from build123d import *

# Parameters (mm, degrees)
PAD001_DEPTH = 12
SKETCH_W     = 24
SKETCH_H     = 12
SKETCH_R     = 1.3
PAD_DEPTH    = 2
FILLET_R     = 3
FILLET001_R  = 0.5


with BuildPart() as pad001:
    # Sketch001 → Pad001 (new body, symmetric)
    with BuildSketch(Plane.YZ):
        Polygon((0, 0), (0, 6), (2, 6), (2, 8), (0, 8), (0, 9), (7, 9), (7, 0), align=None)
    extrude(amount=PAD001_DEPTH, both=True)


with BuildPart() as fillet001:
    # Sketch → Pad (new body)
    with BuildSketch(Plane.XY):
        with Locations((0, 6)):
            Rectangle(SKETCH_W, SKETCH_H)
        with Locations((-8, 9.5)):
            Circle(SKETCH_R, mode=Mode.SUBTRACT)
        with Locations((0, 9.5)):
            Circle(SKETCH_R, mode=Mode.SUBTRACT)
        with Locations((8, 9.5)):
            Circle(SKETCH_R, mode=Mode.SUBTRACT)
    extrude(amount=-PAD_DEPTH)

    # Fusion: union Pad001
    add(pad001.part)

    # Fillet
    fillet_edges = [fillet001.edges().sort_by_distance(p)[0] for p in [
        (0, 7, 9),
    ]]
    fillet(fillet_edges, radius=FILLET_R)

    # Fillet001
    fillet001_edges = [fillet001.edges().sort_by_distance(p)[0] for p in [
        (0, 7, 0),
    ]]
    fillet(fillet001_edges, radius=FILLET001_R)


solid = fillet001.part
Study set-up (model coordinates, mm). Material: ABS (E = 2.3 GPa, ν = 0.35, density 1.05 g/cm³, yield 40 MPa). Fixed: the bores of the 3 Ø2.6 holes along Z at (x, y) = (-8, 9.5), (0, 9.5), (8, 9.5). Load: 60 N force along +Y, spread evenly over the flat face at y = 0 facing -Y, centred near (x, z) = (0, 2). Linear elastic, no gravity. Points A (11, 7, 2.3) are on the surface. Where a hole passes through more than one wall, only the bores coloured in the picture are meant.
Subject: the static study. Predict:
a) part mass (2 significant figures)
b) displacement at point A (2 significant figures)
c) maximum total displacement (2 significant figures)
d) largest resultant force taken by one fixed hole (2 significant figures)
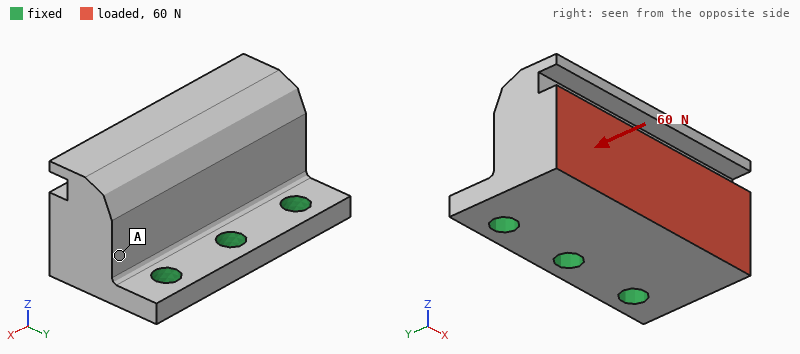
2.0 g
0.042 mm
0.16 mm
20 N
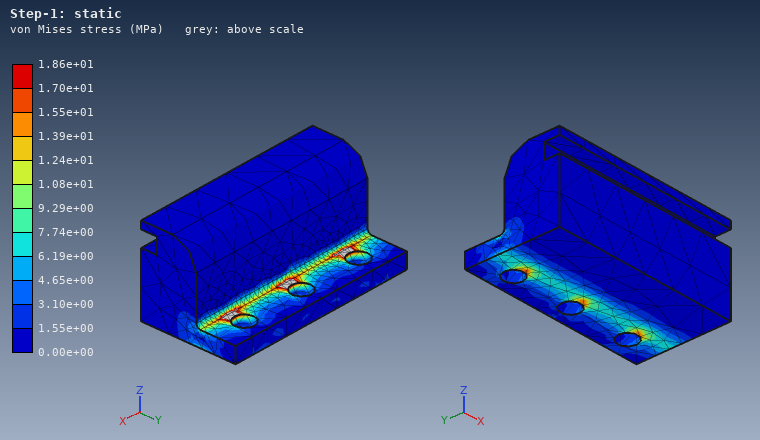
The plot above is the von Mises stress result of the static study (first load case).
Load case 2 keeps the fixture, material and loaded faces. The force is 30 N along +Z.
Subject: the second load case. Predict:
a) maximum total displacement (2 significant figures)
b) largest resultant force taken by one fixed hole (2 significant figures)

0.21 mm
10 N
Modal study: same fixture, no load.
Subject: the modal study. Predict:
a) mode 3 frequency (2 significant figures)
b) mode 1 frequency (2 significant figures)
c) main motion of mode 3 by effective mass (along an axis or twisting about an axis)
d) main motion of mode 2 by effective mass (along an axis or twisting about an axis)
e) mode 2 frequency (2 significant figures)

9000 Hz
2000 Hz
along X
along X
6000 Hz
